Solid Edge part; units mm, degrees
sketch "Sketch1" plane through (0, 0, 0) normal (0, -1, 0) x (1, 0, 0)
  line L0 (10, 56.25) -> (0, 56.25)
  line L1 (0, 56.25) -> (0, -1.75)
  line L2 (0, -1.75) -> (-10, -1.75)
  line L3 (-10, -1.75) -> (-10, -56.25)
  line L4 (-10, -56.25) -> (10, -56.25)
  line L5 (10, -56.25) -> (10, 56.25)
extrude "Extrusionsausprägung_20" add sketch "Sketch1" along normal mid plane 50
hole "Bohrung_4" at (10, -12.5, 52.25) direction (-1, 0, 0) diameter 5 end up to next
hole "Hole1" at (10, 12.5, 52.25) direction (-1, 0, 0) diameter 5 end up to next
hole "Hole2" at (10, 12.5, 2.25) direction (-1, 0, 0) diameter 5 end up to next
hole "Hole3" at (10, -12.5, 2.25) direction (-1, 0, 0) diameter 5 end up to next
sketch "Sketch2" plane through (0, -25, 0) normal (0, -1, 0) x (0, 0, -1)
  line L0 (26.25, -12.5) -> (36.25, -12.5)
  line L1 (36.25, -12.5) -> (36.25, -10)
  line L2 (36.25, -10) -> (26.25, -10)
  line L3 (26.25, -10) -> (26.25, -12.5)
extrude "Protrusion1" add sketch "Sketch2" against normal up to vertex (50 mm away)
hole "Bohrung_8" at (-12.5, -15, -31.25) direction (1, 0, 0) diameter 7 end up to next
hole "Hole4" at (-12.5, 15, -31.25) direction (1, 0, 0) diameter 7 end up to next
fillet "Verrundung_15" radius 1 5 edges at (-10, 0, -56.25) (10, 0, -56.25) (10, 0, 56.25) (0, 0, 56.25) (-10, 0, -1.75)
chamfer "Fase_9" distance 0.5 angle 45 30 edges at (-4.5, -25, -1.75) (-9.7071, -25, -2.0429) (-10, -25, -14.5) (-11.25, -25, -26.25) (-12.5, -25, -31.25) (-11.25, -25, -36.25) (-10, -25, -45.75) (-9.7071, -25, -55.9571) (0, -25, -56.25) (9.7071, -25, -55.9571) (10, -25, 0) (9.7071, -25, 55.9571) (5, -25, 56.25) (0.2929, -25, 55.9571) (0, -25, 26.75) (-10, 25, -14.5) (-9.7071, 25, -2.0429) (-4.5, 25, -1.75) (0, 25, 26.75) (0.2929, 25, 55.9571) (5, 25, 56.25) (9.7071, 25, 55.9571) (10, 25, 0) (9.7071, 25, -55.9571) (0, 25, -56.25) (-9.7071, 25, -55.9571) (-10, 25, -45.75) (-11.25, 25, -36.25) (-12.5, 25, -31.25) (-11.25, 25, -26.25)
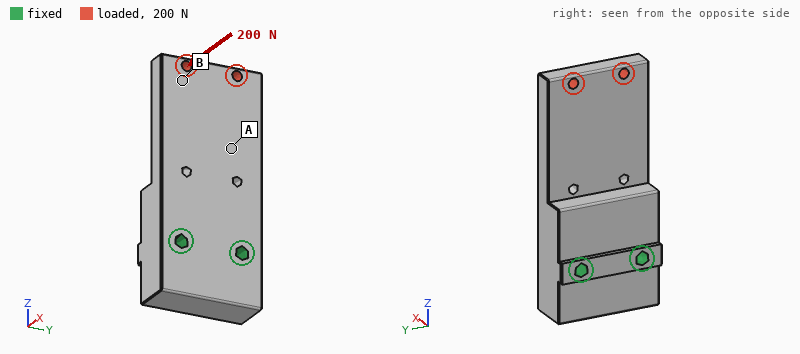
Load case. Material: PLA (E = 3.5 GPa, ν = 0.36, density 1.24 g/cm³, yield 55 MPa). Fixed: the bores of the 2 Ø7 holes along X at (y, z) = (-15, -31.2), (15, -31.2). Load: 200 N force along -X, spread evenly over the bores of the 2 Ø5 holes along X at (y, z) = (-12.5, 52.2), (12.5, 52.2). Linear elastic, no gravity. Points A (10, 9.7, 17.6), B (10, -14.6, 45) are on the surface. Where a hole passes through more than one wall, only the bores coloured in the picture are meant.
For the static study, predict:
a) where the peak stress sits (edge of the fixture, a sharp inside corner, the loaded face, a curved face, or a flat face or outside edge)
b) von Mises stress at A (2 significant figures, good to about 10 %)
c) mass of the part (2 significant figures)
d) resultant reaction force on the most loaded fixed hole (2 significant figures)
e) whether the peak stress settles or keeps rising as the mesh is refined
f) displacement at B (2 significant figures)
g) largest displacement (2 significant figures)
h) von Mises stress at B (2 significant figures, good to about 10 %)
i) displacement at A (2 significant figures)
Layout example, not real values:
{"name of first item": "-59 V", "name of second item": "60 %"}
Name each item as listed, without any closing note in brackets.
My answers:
{"where the peak stress sits": "a sharp inside corner", "von Mises stress at A": "7.7 MPa", "mass of the part": "100 g", "resultant reaction force on the most loaded fixed hole": "100 N", "whether the peak stress settles or keeps rising as the mesh is refined": "keeps rising", "displacement at B": "0.98 mm", "largest displacement": "1.3 mm", "von Mises stress at B": "2.3 MPa", "displacement at A": "0.35 mm"}
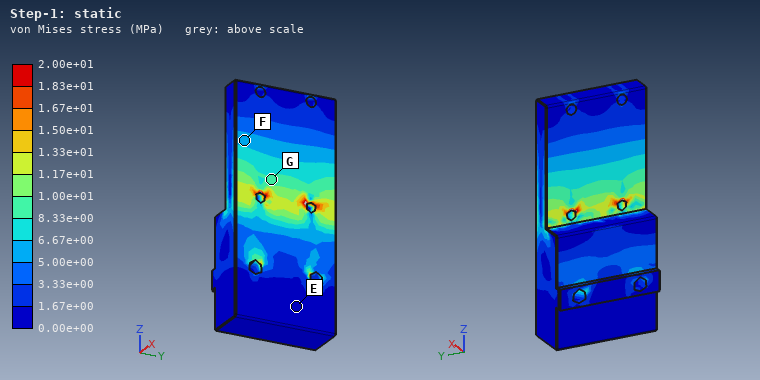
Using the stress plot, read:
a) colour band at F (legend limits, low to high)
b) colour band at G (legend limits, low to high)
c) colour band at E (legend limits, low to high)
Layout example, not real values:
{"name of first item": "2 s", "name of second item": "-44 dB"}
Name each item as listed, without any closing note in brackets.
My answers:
{"colour band at F": "5.00e+00 to 6.67e+00 MPa", "colour band at G": "8.33e+00 to 1.00e+01 MPa", "colour band at E": "0.00e+00 to 1.67e+00 MPa"}
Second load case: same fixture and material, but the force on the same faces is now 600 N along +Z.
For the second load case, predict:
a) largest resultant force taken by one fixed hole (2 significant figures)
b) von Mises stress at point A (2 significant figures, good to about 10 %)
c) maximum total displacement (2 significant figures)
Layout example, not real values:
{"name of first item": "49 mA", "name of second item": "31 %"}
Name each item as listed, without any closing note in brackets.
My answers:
{"largest resultant force taken by one fixed hole": "300 N", "von Mises stress at point A": "1.2 MPa", "maximum total displacement": "70 µm"}
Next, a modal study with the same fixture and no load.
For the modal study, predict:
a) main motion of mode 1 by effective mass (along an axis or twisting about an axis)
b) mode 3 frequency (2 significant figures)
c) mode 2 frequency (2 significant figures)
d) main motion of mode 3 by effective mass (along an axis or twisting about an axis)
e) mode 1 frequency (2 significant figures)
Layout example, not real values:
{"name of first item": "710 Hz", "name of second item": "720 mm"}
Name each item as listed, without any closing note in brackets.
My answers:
{"main motion of mode 1 by effective mass": "along X", "mode 3 frequency": "1700 Hz", "mode 2 frequency": "1600 Hz", "main motion of mode 3 by effective mass": "along Y", "mode 1 frequency": "600 Hz"}
